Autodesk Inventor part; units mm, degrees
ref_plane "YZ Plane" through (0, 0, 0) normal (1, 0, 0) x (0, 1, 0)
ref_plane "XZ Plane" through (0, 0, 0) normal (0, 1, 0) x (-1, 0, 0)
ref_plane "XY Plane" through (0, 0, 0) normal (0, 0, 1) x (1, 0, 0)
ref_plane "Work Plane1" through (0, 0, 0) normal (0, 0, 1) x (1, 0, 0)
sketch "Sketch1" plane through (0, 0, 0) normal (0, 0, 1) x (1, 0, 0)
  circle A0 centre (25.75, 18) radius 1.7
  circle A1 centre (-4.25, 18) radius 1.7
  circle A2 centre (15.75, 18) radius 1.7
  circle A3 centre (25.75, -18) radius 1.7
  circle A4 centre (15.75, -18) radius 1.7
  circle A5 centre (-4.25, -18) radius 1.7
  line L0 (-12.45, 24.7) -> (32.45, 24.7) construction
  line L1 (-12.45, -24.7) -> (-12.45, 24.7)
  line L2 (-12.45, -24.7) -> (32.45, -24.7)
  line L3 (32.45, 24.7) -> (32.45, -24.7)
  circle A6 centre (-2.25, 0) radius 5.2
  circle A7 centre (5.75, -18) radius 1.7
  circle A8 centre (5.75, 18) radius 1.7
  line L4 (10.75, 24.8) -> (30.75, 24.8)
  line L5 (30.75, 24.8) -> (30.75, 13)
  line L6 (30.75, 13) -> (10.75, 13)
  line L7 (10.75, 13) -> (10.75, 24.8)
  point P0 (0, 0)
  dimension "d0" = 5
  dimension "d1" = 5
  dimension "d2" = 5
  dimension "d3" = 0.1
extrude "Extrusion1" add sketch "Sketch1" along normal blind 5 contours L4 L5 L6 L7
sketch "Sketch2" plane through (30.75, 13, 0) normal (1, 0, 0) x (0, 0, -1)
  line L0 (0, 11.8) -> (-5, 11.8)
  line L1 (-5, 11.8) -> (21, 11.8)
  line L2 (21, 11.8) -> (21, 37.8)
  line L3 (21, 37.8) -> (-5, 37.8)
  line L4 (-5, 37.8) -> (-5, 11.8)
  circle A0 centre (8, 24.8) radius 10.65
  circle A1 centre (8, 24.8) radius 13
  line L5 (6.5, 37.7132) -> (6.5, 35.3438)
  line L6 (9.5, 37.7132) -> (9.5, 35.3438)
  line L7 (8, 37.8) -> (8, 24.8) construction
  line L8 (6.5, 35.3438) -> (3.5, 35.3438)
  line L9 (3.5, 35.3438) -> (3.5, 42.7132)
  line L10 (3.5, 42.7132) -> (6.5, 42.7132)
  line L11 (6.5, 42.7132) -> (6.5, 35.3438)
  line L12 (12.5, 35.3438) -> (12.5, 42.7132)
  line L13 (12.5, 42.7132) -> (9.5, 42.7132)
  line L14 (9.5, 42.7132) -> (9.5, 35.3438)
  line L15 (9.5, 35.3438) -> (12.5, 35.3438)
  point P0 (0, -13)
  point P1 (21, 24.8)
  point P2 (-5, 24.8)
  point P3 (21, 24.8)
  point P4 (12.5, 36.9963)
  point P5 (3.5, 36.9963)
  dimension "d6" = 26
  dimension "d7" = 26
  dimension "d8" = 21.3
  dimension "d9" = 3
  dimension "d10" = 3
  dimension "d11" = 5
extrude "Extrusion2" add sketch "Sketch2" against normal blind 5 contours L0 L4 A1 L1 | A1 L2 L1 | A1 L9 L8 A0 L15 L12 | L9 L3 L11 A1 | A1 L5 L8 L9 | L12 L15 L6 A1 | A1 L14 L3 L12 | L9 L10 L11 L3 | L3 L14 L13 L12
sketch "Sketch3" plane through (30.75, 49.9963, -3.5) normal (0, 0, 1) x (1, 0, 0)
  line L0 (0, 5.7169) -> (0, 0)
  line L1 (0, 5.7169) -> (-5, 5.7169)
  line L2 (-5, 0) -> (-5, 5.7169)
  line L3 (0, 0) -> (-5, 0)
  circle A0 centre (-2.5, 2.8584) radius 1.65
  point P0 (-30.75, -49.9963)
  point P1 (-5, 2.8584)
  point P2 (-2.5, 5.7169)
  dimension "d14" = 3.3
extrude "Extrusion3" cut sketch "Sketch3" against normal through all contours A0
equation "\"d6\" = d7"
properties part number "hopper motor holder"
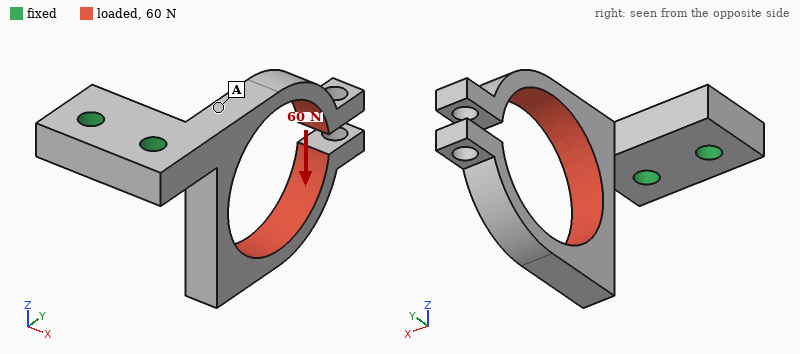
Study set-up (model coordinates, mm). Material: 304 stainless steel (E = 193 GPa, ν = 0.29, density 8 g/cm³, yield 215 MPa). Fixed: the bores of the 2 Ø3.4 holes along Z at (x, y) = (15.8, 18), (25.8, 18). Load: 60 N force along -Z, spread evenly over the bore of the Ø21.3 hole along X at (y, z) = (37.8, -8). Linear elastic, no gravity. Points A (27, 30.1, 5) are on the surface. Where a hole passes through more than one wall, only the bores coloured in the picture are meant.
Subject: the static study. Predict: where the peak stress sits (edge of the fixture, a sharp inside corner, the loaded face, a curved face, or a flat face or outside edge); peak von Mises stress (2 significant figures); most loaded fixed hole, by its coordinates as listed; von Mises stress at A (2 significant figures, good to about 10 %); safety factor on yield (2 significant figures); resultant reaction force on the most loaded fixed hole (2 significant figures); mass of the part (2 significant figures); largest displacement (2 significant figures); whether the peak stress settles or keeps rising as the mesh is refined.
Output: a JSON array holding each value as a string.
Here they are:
["the loaded face", "78 MPa", "(25.8, 18)", "13 MPa", "2.8", "62 N", "19 g", "0.12 mm", "settles"]
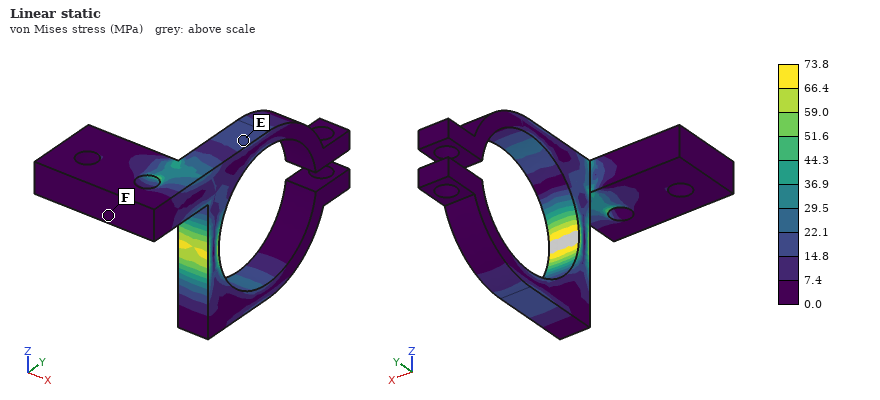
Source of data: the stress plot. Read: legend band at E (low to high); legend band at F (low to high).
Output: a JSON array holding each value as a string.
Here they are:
["14.8 to 22.1 MPa", "0.0 to 7.4 MPa"]
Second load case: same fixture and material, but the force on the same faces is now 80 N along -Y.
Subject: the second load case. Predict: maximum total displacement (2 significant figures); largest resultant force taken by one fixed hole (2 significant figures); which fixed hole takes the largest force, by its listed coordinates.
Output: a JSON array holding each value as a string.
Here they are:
["78 µm", "88 N", "(25.8, 18)"]
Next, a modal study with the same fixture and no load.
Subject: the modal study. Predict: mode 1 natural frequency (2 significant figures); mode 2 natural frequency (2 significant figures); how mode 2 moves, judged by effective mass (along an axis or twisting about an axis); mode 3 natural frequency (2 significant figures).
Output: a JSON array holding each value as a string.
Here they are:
["1300 Hz", "1600 Hz", "along X", "2600 Hz"]
